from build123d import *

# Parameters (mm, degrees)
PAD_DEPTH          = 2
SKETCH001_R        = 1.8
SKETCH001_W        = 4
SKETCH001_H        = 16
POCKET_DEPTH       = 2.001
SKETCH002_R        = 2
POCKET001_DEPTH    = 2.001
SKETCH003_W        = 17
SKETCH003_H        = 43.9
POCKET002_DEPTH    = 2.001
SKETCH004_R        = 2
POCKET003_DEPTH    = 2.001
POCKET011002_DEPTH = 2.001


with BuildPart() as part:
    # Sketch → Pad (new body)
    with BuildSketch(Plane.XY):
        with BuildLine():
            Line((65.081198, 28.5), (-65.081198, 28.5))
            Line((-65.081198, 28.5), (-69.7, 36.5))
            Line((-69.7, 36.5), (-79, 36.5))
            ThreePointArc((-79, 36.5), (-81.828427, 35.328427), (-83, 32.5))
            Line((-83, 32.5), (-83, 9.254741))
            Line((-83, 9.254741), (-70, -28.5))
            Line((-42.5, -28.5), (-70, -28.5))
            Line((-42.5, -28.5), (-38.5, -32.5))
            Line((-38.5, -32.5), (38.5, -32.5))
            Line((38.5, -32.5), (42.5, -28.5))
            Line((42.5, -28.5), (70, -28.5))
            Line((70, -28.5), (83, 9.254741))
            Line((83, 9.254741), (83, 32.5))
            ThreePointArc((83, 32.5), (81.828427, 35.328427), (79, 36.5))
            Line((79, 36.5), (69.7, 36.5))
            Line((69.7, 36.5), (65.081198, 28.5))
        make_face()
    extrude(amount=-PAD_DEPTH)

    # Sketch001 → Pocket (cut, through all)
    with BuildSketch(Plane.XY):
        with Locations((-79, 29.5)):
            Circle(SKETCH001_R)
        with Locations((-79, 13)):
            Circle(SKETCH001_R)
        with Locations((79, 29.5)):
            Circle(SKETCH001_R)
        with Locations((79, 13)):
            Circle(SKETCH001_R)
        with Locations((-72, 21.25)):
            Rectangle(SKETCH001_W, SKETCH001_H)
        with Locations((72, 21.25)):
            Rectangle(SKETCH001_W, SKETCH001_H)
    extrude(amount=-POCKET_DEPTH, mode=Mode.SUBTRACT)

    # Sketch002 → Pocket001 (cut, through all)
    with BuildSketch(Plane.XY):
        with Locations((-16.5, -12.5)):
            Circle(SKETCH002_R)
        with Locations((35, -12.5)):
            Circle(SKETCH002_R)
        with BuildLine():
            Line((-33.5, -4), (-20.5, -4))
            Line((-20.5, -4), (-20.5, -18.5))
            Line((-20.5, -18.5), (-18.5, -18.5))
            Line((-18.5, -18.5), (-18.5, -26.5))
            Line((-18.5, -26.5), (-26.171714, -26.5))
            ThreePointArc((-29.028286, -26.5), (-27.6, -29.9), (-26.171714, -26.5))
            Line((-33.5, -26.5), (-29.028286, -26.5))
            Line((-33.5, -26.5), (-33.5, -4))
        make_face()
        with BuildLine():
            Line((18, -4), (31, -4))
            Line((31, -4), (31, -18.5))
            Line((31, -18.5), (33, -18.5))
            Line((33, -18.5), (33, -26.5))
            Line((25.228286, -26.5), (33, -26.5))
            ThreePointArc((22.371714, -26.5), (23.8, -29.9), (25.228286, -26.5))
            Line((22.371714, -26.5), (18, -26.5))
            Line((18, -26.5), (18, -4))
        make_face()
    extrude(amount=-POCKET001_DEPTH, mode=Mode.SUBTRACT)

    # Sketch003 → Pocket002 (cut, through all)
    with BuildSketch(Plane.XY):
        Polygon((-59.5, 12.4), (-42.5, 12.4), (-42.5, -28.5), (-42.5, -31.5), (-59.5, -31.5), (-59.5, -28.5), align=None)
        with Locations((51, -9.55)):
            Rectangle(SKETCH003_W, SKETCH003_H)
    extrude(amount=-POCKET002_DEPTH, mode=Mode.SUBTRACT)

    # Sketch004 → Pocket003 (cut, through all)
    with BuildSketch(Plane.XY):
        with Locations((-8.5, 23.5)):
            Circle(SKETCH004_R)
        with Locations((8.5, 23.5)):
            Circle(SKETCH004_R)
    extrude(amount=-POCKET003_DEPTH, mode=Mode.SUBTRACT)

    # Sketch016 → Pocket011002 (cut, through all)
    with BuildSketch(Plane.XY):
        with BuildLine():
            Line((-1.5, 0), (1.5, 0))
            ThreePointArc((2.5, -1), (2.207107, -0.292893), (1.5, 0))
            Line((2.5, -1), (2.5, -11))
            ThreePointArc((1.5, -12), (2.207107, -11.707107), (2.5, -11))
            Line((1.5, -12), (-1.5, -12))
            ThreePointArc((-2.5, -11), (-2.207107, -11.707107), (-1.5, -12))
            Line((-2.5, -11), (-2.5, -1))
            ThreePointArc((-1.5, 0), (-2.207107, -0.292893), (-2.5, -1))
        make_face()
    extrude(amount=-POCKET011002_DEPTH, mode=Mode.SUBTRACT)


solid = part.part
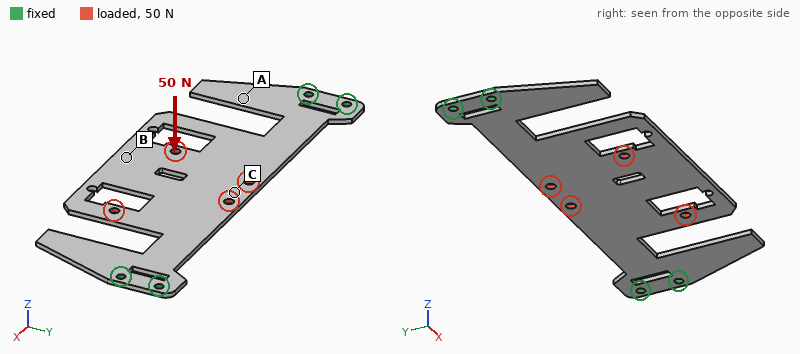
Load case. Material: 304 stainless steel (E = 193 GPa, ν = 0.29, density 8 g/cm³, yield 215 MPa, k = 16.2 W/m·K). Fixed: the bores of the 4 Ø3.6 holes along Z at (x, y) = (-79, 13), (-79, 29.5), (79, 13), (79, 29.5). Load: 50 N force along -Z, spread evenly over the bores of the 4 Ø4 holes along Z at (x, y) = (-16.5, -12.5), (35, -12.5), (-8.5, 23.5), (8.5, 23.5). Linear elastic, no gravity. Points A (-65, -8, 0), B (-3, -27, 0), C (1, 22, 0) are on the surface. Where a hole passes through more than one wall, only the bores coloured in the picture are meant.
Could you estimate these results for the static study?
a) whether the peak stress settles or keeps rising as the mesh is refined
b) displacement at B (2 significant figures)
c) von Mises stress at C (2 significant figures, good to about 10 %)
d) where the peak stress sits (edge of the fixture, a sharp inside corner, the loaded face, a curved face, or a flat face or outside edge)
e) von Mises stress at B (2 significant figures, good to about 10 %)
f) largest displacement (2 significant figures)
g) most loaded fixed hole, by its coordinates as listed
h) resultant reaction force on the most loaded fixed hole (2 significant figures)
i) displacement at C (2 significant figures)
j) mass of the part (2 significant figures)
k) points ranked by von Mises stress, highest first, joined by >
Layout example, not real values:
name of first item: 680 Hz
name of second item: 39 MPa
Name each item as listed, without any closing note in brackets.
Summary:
whether the peak stress settles or keeps rising as the mesh is refined: keeps rising
displacement at B: 0.45 mm
von Mises stress at C: 27 MPa
where the peak stress sits: edge of the fixture
von Mises stress at B: 14 MPa
largest displacement: 0.47 mm
most loaded fixed hole, by its coordinates as listed: (79, 13)
resultant reaction force on the most loaded fixed hole: 33 N
displacement at C: 0.25 mm
mass of the part: 120 g
points ranked by von Mises stress, highest first, joined by >: C > B > A
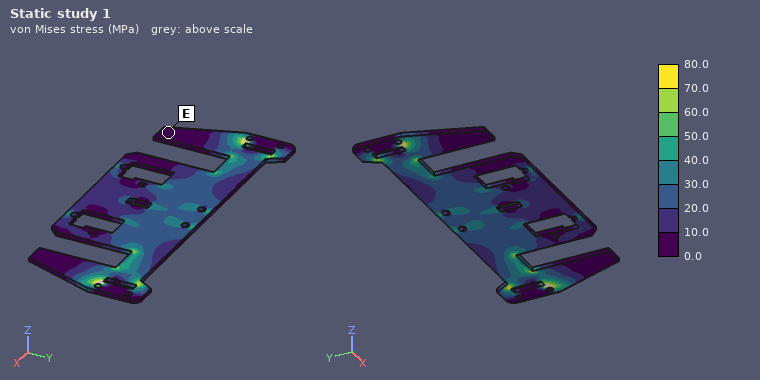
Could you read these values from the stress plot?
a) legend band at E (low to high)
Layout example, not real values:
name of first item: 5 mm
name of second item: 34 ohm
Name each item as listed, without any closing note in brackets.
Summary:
legend band at E: 0.0 to 10.0 MPa
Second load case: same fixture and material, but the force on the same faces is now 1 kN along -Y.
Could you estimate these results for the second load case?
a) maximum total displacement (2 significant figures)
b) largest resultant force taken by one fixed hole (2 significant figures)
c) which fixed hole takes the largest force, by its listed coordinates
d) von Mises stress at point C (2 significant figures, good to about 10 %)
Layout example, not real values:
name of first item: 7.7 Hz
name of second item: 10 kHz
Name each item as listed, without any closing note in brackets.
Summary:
maximum total displacement: 41 µm
largest resultant force taken by one fixed hole: 760 N
which fixed hole takes the largest force, by its listed coordinates: (79, 29.5)
von Mises stress at point C: 14 MPa
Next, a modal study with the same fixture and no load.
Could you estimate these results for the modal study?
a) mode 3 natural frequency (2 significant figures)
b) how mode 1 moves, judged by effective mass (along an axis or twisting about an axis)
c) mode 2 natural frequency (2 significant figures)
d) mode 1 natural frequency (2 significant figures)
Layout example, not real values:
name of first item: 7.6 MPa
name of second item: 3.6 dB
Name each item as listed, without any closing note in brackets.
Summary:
mode 3 natural frequency: 700 Hz
how mode 1 moves, judged by effective mass: along Z
mode 2 natural frequency: 510 Hz
mode 1 natural frequency: 220 Hz
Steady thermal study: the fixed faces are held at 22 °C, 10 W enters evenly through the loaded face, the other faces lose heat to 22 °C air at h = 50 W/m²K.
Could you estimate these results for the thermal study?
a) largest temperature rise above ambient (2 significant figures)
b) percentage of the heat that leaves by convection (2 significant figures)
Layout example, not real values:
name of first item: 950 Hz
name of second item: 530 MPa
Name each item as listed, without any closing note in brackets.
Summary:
largest temperature rise above ambient: 65 K
percentage of the heat that leaves by convection: 99 %
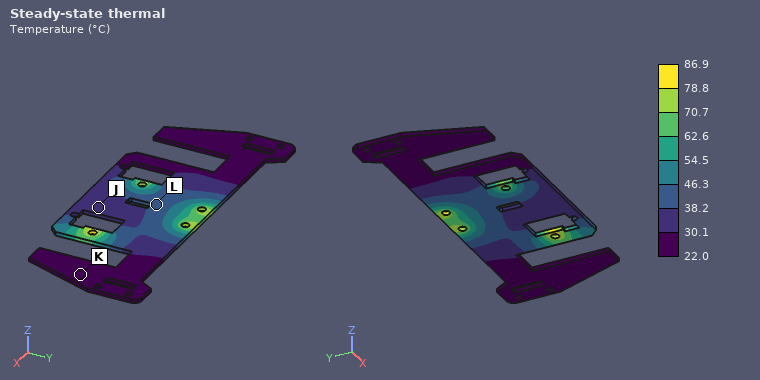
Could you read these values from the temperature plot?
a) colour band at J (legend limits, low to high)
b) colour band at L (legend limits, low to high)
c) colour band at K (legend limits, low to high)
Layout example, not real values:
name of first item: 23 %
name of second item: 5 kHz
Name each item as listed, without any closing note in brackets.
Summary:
colour band at J: 30.1 to 38.2 °C
colour band at L: 38.2 to 46.3 °C
colour band at K: 22.0 to 30.1 °C
